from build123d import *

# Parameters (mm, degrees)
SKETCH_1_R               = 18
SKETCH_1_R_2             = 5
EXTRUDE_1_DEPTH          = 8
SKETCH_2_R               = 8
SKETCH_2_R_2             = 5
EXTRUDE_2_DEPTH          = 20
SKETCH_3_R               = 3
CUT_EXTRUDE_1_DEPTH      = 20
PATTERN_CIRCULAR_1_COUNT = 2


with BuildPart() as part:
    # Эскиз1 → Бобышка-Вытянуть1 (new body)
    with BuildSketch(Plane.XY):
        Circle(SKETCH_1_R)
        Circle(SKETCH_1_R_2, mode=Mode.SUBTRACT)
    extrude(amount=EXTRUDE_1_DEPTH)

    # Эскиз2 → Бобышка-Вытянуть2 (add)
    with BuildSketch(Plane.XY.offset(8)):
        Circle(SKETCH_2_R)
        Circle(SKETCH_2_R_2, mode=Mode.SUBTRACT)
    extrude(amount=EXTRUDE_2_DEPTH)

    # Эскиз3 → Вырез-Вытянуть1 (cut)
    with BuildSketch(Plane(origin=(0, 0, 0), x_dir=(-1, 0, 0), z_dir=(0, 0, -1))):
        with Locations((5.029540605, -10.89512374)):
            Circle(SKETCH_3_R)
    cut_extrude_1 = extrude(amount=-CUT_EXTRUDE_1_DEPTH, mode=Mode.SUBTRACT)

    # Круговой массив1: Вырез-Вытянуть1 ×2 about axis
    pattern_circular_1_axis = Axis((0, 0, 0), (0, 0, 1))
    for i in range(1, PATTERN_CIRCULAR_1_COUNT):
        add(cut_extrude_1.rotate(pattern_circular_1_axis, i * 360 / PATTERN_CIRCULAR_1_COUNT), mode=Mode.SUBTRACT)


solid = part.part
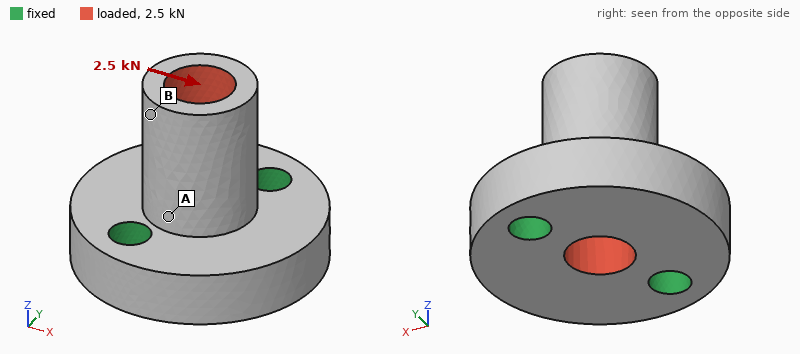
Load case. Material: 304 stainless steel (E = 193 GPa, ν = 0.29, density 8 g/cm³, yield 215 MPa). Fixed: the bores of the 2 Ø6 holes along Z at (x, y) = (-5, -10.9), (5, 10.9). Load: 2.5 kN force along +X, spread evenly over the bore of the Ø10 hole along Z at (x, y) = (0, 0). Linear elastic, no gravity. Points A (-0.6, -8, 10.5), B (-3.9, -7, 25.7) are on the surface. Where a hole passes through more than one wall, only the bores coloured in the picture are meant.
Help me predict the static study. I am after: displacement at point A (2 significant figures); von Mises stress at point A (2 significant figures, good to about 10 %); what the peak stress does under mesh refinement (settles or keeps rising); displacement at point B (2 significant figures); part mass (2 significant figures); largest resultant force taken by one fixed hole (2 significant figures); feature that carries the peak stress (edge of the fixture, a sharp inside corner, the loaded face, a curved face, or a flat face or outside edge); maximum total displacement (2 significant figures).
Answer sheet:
3.1 µm
28 MPa
keeps rising
14 µm
76 g
1.4 kN
edge of the fixture
16 µm
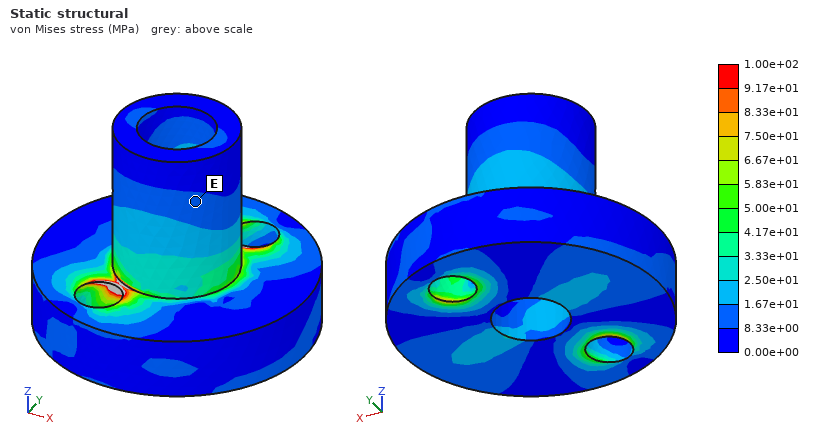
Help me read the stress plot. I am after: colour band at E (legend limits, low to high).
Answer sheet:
8.33e+00 to 1.67e+01 MPa
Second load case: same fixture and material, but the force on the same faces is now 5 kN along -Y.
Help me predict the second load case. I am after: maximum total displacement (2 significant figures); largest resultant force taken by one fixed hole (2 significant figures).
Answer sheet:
23 µm
3.4 kN
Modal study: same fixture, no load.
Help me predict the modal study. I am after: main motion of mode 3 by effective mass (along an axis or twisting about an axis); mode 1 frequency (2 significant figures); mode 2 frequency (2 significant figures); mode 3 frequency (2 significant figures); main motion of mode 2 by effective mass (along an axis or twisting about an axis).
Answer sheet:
along Z
13 kHz
18 kHz
23 kHz
along Y
